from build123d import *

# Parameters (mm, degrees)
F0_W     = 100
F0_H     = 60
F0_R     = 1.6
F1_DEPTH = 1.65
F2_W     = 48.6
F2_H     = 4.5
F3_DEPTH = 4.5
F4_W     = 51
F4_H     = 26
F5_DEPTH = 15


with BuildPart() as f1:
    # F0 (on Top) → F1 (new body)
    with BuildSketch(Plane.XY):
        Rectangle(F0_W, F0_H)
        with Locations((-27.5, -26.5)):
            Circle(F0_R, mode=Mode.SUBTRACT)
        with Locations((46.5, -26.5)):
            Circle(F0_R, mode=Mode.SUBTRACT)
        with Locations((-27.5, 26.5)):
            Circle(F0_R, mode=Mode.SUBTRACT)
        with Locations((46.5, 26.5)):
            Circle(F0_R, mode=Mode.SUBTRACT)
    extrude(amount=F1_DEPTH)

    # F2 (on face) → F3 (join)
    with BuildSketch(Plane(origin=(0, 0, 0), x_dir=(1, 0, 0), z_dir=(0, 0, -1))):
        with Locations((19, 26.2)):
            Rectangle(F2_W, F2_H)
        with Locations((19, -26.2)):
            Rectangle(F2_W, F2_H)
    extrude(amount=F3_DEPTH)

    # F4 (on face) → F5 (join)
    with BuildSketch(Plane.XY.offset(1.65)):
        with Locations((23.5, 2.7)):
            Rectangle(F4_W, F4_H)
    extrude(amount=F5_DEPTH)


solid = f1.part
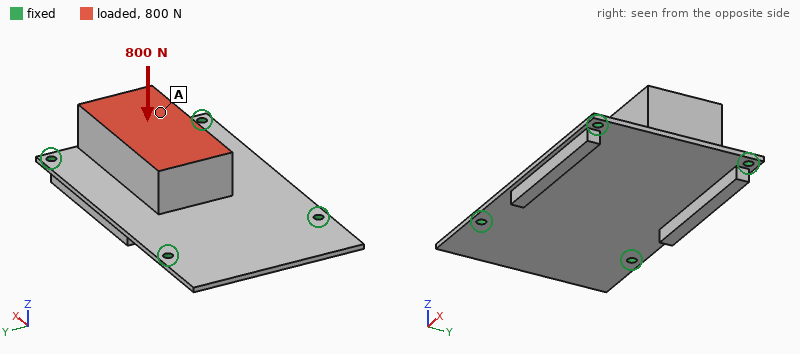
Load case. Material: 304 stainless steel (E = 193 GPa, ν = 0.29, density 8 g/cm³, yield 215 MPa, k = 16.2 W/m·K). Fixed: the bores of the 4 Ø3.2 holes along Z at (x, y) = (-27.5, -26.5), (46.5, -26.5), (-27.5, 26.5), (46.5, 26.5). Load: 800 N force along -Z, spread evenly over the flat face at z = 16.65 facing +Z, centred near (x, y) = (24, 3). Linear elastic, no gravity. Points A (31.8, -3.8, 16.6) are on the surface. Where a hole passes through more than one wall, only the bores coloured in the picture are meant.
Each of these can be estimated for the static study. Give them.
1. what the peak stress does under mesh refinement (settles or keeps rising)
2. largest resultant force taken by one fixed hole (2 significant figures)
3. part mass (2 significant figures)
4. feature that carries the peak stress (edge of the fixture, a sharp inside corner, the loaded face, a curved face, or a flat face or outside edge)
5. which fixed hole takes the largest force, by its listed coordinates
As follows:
keeps rising
360 N
250 g
edge of the fixture
(46.5, 26.5)
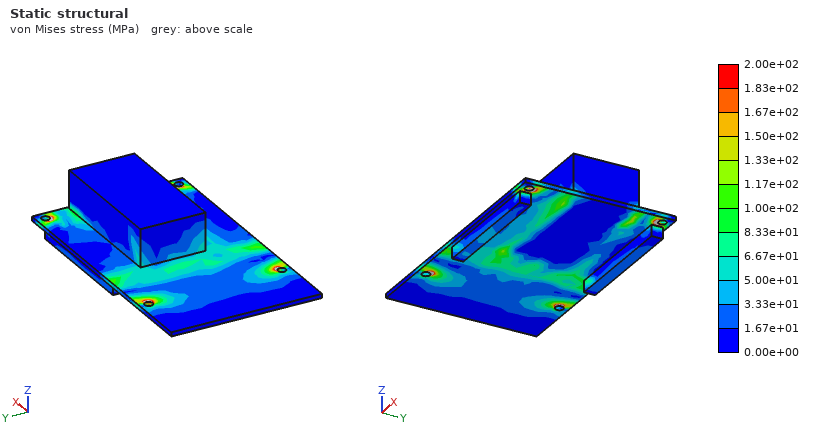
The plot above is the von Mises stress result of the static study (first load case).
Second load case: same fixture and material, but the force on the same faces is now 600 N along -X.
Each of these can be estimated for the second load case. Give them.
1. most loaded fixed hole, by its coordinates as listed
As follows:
(46.5, 26.5)
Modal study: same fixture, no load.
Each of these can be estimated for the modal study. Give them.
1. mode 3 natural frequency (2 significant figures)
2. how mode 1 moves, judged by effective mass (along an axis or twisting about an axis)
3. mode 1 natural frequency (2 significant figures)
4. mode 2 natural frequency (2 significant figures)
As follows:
1900 Hz
along Z
1000 Hz
1800 Hz
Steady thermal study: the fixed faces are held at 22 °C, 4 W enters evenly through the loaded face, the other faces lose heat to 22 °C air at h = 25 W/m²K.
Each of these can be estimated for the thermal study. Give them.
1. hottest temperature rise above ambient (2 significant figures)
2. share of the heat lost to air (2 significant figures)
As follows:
18 K
73 %
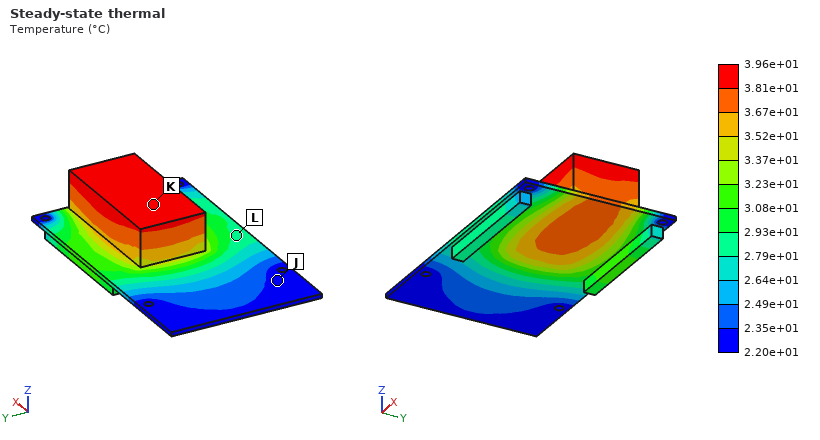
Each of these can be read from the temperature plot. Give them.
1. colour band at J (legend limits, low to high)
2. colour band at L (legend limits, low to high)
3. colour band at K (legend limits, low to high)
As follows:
2.20e+01 to 2.35e+01 °C
2.79e+01 to 2.93e+01 °C
3.81e+01 to 3.96e+01 °C
